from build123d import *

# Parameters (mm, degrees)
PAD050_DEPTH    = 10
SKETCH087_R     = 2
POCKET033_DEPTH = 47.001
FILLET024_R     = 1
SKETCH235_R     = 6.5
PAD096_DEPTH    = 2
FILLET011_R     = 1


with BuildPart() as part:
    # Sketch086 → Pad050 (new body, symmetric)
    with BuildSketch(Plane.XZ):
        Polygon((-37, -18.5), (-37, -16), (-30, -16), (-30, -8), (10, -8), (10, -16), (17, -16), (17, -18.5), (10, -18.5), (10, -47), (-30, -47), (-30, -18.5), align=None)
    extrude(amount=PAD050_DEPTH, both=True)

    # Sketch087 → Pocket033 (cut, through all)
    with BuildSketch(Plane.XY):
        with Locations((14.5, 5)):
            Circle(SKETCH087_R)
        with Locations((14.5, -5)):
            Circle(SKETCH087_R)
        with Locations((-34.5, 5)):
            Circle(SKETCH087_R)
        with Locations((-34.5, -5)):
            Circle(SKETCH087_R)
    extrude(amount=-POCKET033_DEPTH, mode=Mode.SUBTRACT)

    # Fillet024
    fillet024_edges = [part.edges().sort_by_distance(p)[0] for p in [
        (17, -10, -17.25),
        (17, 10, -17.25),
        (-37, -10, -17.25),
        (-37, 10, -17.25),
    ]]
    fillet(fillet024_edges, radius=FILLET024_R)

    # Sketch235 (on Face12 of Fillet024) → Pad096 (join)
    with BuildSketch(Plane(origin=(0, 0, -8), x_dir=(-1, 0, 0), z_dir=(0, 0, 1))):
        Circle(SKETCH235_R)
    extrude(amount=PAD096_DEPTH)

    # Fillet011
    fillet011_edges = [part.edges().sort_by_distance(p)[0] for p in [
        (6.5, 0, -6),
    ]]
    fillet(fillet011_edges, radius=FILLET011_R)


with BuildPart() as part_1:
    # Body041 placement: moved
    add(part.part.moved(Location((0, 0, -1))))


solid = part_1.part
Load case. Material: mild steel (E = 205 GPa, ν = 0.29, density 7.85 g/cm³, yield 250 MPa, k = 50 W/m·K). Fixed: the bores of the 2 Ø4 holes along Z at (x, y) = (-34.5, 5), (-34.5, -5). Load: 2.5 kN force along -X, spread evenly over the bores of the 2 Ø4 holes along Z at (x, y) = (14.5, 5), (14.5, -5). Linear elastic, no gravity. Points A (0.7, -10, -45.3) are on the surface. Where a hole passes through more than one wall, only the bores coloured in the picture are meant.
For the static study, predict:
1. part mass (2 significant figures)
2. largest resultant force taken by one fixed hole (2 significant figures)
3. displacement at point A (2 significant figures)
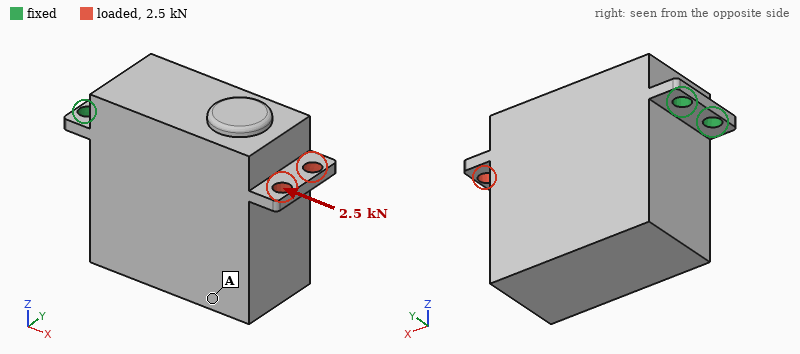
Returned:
250 g
1.3 kN
1.9 µm
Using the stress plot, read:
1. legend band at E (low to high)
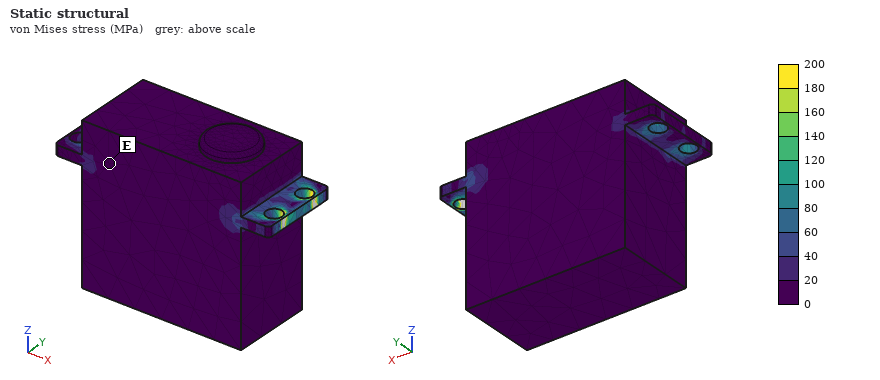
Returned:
0 to 20 MPa
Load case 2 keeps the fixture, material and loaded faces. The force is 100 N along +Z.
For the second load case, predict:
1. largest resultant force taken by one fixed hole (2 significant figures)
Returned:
50 N
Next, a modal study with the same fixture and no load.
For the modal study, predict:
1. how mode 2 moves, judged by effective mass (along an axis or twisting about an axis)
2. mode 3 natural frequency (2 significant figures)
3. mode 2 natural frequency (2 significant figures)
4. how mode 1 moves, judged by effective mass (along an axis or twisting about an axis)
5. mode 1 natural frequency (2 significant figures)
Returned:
along Y
3400 Hz
1900 Hz
along Z
410 Hz
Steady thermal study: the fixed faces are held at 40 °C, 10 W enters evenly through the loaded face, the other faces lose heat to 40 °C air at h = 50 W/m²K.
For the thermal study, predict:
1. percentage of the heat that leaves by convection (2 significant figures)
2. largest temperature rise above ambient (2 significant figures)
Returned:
51 %
57 K
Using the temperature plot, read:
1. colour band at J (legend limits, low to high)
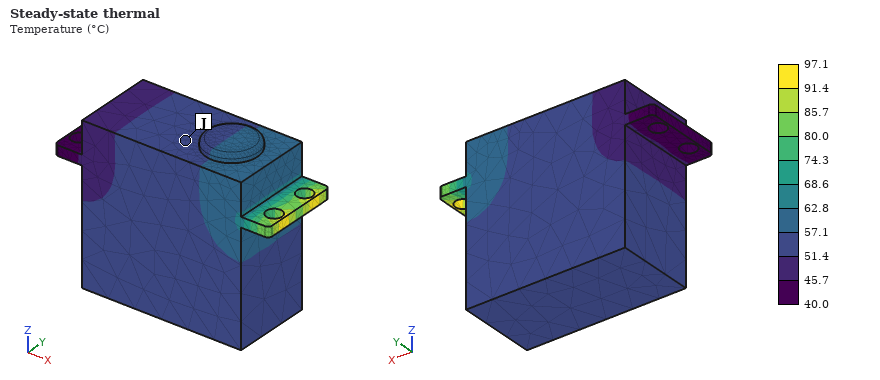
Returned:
51.4 to 57.1 °C
